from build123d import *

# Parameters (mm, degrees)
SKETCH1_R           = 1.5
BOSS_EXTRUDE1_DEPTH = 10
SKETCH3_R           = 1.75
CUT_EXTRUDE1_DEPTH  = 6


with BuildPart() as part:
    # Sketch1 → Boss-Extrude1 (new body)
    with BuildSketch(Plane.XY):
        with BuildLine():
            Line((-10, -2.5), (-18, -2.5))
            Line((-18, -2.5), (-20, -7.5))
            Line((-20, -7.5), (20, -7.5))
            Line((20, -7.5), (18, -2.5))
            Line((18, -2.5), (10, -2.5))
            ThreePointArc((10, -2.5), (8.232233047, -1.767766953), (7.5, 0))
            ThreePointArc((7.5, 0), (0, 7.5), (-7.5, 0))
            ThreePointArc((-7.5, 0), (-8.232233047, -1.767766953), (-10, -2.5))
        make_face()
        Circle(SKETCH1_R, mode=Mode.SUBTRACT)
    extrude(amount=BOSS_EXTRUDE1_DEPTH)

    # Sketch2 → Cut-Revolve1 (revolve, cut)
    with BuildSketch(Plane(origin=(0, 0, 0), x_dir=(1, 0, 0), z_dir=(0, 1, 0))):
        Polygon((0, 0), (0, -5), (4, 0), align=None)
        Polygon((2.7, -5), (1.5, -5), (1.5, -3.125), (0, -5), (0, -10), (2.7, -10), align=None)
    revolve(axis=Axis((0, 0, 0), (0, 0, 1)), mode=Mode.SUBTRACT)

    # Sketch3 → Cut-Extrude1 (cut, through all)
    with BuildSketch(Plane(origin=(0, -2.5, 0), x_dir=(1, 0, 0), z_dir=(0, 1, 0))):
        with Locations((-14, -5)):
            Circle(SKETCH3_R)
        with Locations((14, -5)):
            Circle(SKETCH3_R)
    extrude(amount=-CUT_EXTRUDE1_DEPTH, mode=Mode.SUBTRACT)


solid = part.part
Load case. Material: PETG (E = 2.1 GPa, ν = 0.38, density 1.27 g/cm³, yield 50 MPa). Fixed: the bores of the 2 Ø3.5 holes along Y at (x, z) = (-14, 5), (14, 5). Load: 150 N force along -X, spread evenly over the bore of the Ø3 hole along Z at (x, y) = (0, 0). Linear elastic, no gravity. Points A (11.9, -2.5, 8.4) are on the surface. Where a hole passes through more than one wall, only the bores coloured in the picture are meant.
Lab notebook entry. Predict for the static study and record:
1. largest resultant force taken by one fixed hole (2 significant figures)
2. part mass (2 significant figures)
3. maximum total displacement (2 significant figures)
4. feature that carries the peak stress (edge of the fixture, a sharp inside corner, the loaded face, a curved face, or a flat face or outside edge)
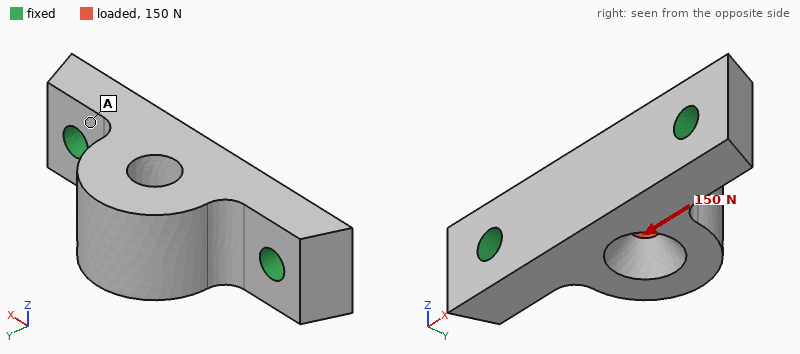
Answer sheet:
82 N
3.7 g
26 µm
the loaded face
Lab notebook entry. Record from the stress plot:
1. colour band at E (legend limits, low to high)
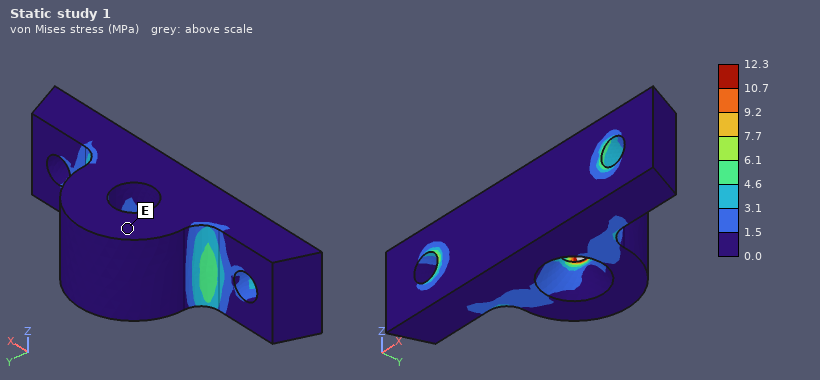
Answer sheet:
0.0 to 1.5 MPa
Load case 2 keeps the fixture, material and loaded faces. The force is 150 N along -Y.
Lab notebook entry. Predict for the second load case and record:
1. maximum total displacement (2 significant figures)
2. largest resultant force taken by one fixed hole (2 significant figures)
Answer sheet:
49 µm
82 N
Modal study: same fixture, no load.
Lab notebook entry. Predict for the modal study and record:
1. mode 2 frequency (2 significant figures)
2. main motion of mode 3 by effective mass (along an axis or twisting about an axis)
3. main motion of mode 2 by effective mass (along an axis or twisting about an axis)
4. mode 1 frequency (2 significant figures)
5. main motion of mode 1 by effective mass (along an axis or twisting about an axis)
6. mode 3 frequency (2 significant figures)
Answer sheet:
7100 Hz
along Z
along Y
3900 Hz
along Z
9100 Hz
